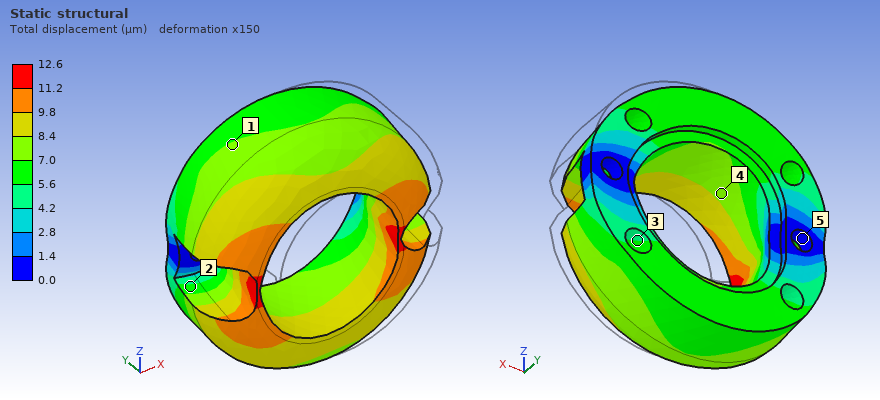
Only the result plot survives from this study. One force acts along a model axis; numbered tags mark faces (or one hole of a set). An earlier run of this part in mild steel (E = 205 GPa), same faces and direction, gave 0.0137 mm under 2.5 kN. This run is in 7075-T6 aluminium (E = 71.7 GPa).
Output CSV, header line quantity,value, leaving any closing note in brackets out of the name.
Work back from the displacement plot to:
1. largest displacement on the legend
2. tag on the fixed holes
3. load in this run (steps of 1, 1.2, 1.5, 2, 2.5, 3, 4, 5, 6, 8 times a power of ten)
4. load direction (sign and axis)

quantity,value
largest displacement on the legend,12.6 µm
tag on the fixed holes,5
load in this run,800 N
load direction,-X
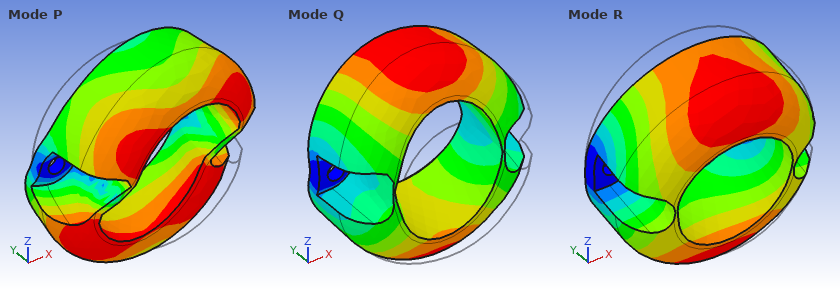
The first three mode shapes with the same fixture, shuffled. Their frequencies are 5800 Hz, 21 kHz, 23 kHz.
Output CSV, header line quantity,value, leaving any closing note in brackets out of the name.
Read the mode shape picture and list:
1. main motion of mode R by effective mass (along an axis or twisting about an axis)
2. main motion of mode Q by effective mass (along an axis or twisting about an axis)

quantity,value
main motion of mode R by effective mass,along Z
main motion of mode Q by effective mass,along Y
